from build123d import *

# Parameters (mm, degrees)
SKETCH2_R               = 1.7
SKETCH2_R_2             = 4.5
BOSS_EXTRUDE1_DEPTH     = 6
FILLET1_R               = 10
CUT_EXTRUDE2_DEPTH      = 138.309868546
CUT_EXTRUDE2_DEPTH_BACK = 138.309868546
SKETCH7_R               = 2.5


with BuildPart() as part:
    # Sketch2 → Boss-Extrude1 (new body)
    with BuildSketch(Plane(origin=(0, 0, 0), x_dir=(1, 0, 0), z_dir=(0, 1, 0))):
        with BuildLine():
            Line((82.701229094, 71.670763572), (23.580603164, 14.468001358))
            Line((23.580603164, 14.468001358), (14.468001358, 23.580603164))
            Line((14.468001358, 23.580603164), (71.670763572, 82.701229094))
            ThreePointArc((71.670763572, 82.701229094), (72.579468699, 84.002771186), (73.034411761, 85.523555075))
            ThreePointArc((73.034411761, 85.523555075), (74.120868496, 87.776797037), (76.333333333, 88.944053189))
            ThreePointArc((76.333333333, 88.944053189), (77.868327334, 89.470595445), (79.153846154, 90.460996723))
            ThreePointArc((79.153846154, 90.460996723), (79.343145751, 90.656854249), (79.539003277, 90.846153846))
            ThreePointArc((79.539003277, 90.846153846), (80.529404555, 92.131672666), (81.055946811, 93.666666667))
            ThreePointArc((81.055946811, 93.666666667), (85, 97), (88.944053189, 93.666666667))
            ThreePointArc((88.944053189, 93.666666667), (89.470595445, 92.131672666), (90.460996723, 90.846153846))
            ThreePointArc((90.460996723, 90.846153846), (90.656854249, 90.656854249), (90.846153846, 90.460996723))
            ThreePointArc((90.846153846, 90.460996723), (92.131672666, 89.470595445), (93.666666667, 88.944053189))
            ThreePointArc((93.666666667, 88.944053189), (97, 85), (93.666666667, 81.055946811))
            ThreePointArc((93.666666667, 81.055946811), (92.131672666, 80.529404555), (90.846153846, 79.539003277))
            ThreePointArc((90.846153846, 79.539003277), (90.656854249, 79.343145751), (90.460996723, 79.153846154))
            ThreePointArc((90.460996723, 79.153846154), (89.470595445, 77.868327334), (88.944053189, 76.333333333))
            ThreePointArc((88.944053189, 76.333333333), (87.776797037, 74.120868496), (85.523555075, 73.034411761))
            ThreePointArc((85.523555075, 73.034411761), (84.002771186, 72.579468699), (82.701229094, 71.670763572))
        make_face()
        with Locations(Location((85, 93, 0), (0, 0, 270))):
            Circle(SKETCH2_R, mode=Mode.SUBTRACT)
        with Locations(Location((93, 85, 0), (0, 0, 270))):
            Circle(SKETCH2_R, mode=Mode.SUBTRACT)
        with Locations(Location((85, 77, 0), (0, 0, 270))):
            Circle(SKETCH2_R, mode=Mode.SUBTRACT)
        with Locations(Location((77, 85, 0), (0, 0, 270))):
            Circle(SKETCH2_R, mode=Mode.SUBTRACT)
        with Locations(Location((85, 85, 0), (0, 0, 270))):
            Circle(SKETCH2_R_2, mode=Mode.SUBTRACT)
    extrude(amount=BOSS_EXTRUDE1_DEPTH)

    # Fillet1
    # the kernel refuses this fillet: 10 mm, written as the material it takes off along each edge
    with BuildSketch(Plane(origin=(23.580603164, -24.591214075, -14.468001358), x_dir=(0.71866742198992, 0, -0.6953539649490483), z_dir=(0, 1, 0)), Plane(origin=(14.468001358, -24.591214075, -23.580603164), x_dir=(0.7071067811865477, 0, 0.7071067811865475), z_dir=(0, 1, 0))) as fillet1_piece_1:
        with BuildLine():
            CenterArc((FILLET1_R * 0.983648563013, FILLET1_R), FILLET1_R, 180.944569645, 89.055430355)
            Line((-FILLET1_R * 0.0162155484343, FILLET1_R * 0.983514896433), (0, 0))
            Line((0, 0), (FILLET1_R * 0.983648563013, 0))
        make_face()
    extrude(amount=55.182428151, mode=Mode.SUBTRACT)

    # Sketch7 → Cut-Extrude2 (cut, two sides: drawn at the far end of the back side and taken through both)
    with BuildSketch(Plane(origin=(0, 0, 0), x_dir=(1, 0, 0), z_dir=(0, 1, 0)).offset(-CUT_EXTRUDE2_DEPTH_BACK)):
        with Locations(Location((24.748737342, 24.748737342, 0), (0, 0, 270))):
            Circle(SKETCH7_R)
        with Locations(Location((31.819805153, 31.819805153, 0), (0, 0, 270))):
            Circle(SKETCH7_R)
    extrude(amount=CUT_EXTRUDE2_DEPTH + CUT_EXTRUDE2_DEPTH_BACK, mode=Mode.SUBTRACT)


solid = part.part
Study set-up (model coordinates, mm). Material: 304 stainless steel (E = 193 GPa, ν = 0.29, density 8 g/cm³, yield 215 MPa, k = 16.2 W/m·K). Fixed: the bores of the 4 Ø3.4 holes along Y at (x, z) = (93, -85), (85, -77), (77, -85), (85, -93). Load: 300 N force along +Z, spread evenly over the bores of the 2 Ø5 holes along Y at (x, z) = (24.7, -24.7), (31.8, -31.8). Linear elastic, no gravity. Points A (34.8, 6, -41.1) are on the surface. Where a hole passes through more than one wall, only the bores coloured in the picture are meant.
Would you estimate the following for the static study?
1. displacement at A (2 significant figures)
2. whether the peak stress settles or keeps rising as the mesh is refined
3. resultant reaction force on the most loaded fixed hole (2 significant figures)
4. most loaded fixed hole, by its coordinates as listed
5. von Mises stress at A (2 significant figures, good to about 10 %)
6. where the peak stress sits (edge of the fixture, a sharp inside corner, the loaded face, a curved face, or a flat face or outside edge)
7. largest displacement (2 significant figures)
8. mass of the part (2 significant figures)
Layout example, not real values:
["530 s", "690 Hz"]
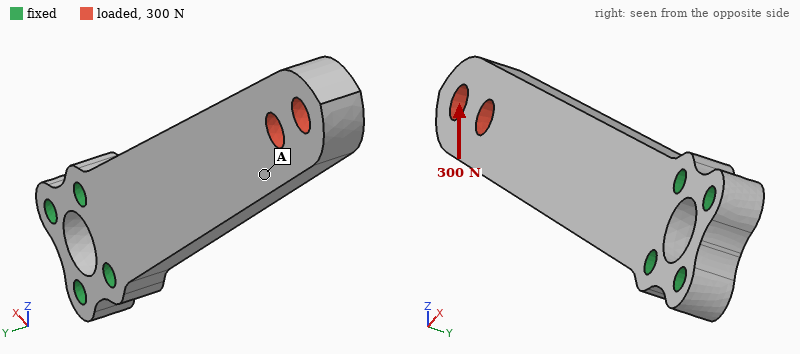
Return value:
["0.061 mm", "keeps rising", "1.4 kN", "(77, -85)", "13 MPa", "edge of the fixture", "0.11 mm", "64 g"]
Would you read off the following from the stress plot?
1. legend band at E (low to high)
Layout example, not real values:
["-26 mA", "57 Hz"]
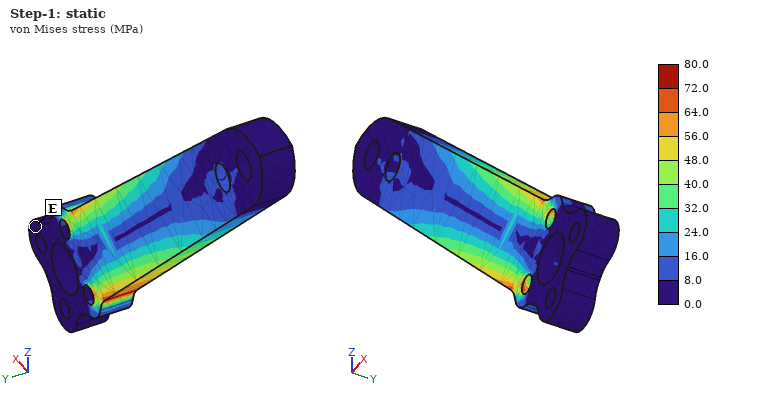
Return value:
["0.0 to 8.0 MPa"]
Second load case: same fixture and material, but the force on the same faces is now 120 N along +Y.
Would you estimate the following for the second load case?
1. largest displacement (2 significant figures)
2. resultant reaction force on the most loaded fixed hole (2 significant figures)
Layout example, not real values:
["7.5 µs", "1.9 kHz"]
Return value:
["0.39 mm", "74 N"]
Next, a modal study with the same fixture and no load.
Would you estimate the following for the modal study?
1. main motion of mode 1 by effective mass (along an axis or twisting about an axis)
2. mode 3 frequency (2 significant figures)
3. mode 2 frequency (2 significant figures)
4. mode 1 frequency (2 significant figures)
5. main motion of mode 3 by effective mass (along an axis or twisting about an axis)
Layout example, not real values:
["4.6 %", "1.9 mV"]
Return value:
["along Y", "4200 Hz", "1900 Hz", "750 Hz", "along Y"]
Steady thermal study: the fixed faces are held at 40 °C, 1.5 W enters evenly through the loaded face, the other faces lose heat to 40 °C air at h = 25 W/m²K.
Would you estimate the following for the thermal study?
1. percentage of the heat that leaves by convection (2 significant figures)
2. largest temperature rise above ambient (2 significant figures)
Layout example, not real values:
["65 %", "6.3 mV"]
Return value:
["78 %", "33 K"]
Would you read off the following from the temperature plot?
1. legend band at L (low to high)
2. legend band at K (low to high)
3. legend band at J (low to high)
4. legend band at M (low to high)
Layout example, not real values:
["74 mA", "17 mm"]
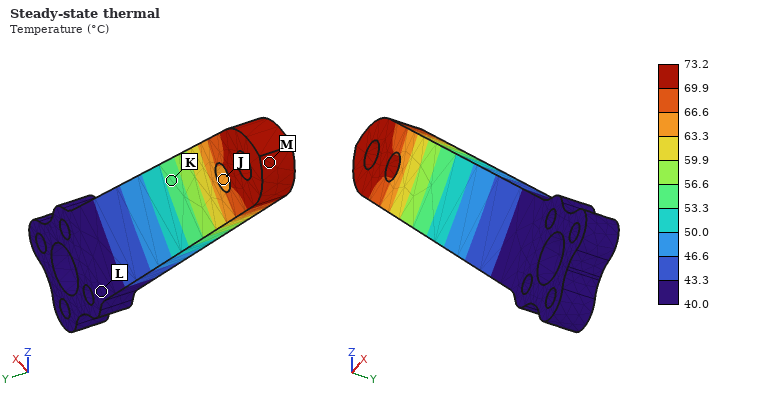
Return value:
["40.0 to 43.3 °C", "53.3 to 56.6 °C", "63.3 to 66.6 °C", "69.9 to 73.2 °C"]
